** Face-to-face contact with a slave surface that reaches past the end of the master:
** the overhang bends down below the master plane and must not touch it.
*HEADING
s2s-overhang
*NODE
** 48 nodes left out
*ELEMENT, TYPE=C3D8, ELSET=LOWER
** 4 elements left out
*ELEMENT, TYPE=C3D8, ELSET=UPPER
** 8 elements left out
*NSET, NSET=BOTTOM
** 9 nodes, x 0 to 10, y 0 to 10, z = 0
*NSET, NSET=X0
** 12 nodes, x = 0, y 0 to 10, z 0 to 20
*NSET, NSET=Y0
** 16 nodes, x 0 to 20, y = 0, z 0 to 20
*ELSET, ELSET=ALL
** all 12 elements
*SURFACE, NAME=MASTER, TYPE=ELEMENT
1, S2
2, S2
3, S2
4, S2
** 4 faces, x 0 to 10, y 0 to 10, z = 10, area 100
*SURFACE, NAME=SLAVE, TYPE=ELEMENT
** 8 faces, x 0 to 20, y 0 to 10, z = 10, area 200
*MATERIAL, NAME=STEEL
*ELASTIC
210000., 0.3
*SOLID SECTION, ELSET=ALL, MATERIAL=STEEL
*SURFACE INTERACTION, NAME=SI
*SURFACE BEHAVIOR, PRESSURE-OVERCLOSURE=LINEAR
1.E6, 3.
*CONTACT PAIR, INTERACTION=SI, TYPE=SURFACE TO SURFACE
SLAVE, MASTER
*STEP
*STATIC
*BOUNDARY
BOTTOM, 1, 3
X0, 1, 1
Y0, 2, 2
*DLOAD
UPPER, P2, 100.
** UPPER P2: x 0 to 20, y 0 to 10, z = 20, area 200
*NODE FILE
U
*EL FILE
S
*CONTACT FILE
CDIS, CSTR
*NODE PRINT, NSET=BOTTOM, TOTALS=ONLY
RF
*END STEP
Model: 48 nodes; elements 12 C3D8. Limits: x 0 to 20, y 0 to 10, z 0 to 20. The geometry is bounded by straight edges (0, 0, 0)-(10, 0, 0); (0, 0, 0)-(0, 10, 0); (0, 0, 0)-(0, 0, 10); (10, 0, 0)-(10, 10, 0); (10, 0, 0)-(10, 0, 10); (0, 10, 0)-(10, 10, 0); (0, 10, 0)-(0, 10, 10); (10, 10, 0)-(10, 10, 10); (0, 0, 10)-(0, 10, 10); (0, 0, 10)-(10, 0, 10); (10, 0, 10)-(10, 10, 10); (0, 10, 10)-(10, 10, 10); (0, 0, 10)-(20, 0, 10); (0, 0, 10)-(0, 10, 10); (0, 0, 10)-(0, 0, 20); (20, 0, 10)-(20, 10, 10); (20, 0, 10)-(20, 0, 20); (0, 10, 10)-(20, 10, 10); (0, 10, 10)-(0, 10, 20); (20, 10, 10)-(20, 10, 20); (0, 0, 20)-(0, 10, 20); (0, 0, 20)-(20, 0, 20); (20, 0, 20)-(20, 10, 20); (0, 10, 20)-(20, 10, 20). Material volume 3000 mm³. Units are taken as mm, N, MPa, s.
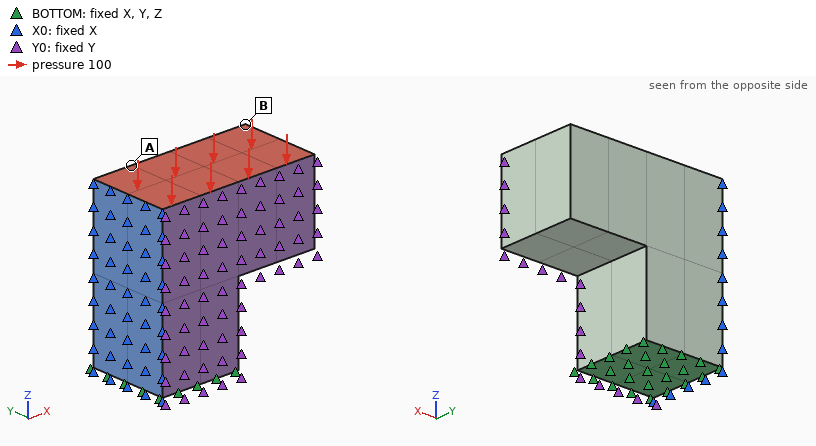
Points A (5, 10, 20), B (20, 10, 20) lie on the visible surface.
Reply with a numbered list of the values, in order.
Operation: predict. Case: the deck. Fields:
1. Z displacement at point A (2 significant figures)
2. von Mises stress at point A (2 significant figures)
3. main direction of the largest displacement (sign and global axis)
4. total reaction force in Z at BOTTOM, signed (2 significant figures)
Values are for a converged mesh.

1. -0.011 mm
2. 450 MPa
3. -Z
4. 20000 N
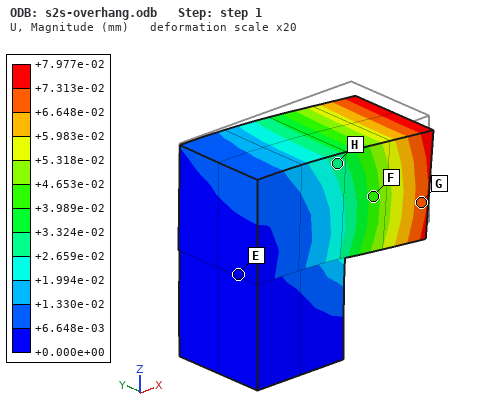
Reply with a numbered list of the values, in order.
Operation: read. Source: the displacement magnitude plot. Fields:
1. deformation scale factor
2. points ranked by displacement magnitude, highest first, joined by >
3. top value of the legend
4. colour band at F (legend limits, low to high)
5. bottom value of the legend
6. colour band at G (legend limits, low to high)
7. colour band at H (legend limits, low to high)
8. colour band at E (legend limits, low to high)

1. 20
2. G > F > H > E
3. +7.977e-02 mm
4. +3.989e-02 to +4.653e-02 mm
5. +0.000e+00 mm
6. +6.648e-02 to +7.313e-02 mm
7. +2.659e-02 to +3.324e-02 mm
8. +0.000e+00 to +6.648e-03 mm
